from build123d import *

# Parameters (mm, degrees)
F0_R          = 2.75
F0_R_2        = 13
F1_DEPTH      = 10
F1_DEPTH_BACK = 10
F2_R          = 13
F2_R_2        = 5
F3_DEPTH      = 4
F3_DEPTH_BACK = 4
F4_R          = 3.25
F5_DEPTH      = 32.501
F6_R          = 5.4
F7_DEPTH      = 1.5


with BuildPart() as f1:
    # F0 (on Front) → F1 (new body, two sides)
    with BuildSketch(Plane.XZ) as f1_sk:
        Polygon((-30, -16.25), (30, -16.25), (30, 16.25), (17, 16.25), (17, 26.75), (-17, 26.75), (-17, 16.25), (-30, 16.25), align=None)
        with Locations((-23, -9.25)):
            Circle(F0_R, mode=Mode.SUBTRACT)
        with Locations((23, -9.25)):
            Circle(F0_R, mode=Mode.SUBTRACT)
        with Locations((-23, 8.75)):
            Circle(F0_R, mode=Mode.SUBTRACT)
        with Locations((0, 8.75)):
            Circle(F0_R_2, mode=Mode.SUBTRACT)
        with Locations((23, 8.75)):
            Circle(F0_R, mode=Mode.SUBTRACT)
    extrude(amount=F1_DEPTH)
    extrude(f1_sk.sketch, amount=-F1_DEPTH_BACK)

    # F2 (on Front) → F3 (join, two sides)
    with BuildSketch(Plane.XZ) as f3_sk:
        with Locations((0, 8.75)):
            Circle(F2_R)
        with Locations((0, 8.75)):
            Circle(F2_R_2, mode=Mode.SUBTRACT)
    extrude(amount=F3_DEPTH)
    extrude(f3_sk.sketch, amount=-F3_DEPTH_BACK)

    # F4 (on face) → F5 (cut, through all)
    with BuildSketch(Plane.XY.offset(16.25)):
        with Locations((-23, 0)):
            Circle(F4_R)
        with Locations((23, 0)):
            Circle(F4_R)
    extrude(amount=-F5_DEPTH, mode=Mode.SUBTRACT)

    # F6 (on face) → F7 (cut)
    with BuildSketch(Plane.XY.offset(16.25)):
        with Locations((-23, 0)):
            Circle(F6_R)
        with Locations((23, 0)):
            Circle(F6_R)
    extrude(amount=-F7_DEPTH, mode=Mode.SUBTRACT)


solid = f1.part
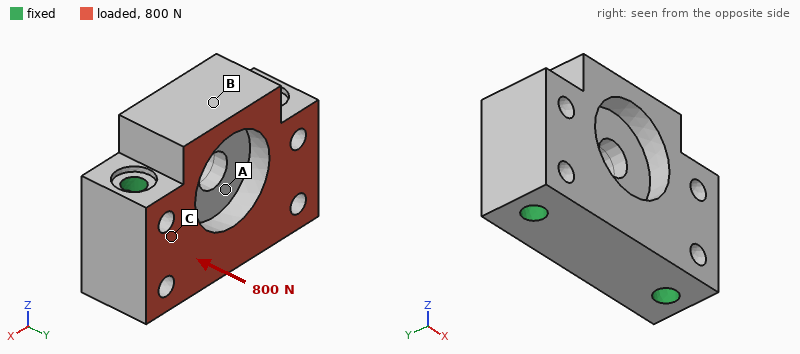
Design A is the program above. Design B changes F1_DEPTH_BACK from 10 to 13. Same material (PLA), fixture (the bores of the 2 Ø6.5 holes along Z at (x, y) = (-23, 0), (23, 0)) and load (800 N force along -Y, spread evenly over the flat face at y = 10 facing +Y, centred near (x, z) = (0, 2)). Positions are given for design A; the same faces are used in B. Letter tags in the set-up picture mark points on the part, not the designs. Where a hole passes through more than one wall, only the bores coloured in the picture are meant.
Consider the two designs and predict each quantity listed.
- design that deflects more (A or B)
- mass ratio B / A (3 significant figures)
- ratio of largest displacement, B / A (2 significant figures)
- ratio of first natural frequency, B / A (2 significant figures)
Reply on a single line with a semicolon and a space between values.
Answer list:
A; 1.14; 0.88; 1.0
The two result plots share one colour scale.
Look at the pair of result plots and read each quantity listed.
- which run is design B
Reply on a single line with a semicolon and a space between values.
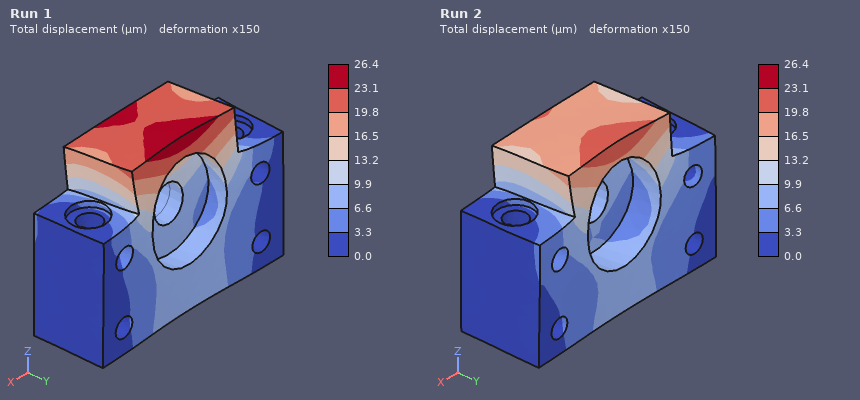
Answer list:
Run 2
